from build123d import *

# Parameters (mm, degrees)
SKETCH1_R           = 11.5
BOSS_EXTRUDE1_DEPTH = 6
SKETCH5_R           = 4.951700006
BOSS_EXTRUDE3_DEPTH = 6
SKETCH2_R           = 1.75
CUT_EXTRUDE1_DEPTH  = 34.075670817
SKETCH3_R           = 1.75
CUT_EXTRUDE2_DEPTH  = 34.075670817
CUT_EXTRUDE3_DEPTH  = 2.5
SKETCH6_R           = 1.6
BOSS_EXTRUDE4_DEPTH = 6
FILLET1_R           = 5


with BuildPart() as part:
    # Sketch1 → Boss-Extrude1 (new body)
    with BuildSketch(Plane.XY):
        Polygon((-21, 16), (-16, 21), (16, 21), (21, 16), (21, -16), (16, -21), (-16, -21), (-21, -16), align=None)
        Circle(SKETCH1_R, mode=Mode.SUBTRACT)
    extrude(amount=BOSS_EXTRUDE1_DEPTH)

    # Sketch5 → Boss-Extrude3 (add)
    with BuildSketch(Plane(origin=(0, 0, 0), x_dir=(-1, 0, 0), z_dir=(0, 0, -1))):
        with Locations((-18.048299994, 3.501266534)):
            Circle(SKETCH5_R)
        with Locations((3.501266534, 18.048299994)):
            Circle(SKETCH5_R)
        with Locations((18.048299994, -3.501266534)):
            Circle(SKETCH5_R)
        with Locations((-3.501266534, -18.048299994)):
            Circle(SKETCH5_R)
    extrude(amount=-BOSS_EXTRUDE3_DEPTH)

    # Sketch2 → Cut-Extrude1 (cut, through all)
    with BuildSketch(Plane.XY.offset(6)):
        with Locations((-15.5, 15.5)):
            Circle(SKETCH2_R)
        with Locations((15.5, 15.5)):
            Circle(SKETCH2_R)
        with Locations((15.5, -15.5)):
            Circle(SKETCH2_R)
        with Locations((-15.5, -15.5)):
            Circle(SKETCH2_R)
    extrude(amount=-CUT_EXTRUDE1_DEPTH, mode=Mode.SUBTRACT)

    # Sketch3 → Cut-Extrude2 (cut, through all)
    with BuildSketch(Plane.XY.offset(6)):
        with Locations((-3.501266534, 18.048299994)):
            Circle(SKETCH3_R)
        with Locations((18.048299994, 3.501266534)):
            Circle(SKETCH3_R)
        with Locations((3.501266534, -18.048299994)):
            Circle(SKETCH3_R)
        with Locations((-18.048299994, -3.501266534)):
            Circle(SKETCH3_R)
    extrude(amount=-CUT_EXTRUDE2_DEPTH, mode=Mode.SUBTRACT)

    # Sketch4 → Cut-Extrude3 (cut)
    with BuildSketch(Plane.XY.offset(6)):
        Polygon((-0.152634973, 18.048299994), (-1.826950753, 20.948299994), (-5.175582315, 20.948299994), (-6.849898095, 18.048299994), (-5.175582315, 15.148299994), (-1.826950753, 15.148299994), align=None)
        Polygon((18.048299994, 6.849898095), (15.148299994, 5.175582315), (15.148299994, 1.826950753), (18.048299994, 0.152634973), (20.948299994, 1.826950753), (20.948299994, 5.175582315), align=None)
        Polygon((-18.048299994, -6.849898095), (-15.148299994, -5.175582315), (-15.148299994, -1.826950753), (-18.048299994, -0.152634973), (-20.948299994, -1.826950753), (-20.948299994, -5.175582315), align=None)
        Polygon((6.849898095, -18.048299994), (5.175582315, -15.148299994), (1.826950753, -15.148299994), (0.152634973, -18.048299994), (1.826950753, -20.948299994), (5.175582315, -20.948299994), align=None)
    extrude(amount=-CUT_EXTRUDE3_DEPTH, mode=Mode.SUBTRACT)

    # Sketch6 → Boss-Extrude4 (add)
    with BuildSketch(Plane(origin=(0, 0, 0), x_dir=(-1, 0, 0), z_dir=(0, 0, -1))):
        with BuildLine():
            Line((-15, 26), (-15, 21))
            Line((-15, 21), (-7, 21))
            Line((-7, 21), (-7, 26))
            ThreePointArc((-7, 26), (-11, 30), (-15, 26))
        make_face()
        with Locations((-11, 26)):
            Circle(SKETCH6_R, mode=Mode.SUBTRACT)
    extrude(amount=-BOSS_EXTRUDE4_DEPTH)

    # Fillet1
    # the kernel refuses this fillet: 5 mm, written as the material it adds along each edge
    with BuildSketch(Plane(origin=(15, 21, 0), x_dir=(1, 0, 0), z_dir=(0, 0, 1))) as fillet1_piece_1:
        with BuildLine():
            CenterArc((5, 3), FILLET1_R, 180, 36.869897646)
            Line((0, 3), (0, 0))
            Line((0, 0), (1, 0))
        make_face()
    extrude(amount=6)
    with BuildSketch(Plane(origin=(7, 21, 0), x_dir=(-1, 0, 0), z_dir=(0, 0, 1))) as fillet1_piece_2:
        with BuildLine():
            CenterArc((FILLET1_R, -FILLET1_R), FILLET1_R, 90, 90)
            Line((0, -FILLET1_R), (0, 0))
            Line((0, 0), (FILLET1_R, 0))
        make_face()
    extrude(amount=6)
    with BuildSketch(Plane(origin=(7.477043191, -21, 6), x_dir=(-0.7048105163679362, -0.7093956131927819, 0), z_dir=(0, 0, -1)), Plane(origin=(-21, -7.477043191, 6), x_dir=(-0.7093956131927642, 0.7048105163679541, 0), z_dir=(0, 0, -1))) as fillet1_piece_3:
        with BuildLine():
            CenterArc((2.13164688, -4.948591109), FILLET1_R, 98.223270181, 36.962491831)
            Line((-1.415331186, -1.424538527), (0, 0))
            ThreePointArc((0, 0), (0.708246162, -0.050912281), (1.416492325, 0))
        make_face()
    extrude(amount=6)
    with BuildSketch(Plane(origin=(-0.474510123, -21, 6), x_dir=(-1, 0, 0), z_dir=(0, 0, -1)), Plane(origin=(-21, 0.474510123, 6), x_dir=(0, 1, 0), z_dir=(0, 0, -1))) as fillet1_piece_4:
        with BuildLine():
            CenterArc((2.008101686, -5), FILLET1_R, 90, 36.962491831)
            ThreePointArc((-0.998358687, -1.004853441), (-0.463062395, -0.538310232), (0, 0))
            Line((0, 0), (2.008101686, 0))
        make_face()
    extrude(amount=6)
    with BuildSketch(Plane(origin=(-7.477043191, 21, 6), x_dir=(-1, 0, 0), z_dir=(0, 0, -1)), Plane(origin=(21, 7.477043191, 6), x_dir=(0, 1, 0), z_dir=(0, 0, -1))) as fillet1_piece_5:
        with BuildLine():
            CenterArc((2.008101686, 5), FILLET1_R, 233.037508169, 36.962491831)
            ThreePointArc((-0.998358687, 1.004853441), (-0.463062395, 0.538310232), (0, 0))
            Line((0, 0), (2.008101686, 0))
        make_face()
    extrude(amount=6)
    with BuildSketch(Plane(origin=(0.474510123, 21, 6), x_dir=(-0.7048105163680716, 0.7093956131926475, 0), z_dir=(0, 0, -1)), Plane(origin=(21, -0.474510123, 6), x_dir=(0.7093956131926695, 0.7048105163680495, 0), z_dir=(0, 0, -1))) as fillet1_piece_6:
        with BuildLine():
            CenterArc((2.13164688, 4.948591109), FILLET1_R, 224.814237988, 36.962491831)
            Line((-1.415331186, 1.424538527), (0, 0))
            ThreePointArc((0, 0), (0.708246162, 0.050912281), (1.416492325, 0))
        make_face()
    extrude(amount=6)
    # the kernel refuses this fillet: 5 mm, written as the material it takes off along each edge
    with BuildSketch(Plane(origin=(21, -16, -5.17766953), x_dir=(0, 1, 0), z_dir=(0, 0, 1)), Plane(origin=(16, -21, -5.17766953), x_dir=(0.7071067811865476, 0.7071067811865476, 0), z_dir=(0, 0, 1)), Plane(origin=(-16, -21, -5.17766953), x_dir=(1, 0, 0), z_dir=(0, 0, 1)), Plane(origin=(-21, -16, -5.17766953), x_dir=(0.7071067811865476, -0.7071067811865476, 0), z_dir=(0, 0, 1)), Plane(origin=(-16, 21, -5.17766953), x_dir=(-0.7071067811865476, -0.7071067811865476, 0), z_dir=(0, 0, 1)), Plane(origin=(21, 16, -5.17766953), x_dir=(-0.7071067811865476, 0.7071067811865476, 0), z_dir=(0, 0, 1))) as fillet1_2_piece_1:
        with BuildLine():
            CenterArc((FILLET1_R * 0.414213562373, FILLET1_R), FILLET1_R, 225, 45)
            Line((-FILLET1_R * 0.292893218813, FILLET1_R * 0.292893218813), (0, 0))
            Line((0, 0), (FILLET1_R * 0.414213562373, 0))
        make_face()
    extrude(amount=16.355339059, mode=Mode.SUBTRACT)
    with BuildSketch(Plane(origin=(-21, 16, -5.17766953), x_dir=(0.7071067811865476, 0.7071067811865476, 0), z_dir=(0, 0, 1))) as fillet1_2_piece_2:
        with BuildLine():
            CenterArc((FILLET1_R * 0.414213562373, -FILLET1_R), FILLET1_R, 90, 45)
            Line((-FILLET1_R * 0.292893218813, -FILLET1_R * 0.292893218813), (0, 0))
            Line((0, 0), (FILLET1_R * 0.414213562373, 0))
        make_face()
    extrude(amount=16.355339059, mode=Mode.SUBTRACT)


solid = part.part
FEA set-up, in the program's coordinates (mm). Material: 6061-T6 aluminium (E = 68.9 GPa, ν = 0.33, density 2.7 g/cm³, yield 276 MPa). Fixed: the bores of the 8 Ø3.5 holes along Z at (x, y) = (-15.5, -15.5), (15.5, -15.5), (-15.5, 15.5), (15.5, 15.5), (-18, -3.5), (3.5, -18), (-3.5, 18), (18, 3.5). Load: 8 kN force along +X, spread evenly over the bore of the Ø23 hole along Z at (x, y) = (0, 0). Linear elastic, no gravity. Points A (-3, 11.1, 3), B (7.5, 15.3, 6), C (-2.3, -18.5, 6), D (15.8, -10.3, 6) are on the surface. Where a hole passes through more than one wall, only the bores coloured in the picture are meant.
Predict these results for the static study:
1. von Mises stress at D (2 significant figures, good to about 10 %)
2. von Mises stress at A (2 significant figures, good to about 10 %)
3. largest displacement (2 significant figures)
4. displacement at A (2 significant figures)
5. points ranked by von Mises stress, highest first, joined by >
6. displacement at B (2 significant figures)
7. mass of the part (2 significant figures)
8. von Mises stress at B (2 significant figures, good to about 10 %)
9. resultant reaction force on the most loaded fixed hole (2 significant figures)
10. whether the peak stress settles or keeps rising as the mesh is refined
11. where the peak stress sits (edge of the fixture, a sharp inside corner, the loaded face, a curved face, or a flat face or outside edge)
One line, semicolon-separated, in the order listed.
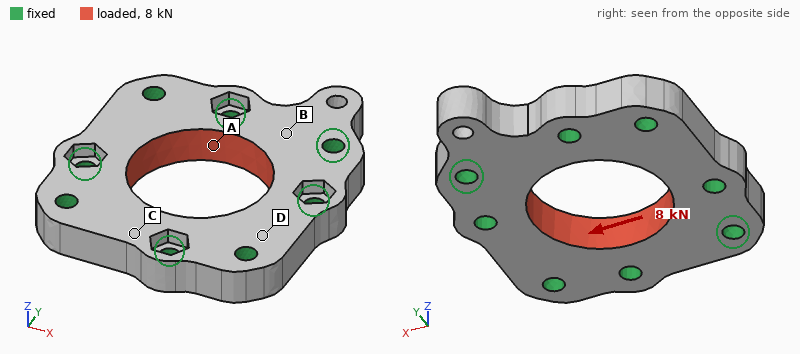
21 MPa; 31 MPa; 6.3 µm; 3.8 µm; A > D > B > C; 1.4 µm; 21 g; 13 MPa; 1.4 kN; keeps rising; edge of the fixture
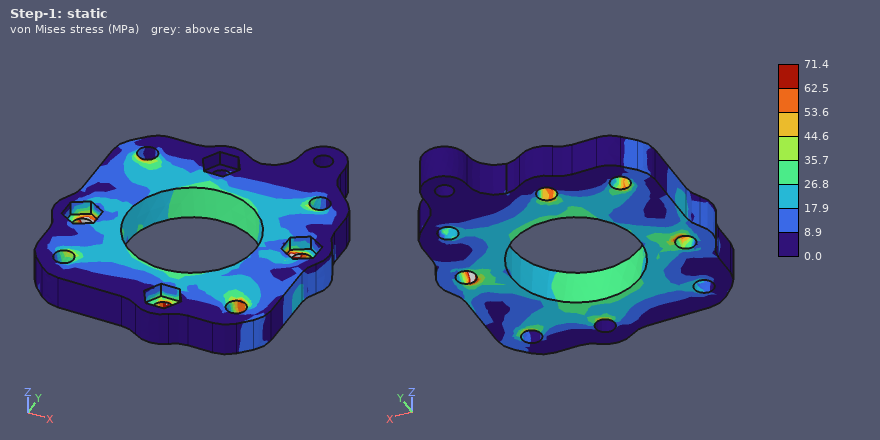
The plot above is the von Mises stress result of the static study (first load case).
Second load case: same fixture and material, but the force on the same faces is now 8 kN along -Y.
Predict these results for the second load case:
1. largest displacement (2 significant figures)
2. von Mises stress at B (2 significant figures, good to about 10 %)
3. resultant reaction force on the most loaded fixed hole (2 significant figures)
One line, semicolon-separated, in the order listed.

6.3 µm; 17 MPa; 1.4 kN
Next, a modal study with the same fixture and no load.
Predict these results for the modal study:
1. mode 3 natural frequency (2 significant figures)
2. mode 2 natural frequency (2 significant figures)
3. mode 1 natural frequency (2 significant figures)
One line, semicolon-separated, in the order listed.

46 kHz; 46 kHz; 28 kHz
